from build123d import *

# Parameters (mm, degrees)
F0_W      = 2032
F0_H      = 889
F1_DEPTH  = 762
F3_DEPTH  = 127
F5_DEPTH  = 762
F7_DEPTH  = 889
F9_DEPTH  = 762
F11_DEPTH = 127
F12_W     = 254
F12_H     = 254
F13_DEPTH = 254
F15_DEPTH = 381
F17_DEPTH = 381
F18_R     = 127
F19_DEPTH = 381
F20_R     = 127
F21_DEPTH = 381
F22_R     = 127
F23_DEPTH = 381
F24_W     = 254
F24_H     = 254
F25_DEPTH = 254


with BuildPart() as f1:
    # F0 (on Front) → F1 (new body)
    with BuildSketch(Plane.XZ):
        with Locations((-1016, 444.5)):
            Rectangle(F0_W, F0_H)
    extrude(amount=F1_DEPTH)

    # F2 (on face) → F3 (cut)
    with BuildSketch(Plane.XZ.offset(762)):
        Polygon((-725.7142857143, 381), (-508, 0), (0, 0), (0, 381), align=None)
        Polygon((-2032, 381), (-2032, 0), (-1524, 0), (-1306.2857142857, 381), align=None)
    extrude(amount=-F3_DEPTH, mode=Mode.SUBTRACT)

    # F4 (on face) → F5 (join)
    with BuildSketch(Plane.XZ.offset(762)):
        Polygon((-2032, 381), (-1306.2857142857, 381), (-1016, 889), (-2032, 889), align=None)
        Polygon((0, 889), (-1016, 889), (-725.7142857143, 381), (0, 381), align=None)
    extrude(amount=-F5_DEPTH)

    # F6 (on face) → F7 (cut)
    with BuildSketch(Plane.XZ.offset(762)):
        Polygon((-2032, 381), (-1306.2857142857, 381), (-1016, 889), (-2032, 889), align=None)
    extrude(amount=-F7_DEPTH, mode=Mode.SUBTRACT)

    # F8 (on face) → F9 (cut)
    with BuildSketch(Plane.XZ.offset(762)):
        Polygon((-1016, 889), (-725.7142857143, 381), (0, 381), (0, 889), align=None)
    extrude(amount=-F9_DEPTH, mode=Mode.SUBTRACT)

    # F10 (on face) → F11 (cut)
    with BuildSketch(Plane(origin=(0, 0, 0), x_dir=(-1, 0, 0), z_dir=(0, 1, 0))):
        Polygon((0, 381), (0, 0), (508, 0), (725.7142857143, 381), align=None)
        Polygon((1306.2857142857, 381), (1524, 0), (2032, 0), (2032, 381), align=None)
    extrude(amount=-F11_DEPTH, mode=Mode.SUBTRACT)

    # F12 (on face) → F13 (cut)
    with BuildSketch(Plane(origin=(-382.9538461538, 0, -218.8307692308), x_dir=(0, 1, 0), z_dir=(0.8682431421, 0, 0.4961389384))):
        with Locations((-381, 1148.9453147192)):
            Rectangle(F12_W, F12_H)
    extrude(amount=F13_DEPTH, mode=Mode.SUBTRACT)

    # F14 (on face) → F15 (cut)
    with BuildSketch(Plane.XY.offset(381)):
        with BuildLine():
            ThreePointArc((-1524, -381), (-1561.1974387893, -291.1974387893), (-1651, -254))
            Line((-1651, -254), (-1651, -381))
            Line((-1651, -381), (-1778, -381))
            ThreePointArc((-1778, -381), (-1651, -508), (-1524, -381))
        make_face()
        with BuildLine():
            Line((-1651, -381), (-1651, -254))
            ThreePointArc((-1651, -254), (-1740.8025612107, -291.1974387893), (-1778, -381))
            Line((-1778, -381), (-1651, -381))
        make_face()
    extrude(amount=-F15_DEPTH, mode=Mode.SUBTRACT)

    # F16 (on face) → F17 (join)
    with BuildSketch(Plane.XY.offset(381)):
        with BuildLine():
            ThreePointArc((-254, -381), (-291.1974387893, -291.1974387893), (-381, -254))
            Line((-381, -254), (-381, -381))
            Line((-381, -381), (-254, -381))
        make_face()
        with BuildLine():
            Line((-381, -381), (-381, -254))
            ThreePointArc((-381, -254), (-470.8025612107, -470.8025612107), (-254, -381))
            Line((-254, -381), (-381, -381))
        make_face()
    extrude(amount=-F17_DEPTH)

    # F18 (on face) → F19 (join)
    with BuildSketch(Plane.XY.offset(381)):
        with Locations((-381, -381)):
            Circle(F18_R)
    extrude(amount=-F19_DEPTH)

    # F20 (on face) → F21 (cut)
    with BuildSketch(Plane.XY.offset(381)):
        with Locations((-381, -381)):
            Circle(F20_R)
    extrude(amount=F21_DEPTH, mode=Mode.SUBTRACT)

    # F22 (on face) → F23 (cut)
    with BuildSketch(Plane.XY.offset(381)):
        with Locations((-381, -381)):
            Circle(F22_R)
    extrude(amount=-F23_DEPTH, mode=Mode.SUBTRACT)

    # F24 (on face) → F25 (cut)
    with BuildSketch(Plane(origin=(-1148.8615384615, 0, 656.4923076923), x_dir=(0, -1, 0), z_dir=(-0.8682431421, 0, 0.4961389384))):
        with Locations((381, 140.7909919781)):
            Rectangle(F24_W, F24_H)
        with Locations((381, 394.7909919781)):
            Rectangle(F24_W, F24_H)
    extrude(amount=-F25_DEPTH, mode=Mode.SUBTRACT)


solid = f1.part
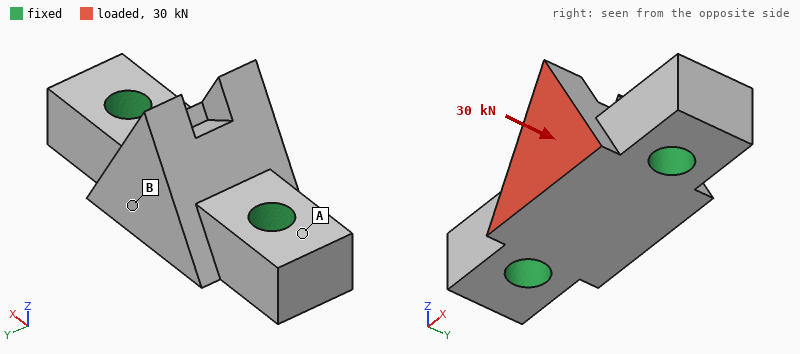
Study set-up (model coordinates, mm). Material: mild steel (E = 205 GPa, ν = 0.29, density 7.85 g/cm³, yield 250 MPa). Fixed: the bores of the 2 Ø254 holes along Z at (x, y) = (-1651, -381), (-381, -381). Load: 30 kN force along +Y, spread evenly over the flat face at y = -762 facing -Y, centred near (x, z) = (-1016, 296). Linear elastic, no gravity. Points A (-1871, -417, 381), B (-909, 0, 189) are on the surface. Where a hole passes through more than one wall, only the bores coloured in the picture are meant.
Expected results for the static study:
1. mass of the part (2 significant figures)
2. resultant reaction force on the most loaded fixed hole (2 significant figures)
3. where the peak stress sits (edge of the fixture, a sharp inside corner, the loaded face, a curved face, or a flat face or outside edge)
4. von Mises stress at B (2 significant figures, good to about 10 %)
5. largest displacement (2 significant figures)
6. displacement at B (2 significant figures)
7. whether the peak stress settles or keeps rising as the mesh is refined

4200 kg
15 kN
edge of the fixture
0.10 MPa
2.0 µm
0.59 µm
keeps rising
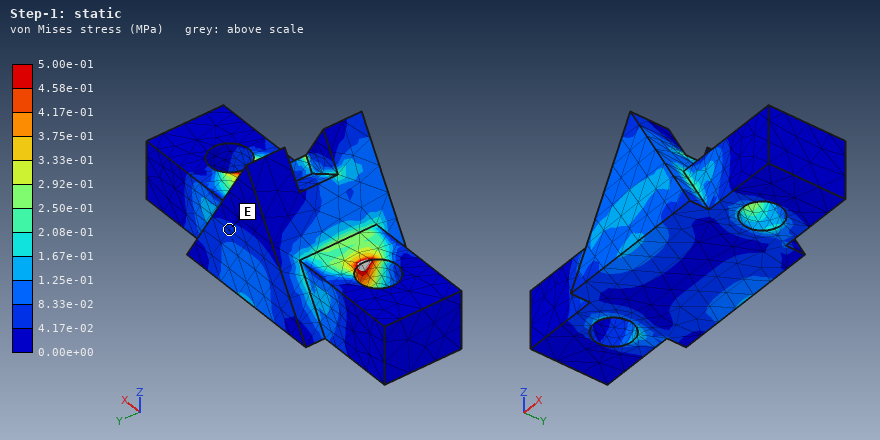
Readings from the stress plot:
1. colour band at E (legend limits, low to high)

4.17e-02 to 8.33e-02 MPa
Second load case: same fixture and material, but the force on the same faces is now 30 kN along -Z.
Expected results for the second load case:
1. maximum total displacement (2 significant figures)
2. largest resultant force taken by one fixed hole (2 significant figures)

4.2 µm
15 kN
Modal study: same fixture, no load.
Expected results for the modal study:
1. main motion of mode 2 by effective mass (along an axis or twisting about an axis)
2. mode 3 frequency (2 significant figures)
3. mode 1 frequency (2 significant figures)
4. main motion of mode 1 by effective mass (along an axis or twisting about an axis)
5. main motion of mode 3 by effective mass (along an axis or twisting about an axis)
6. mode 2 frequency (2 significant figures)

along Z
950 Hz
510 Hz
along Y
along Y
770 Hz
